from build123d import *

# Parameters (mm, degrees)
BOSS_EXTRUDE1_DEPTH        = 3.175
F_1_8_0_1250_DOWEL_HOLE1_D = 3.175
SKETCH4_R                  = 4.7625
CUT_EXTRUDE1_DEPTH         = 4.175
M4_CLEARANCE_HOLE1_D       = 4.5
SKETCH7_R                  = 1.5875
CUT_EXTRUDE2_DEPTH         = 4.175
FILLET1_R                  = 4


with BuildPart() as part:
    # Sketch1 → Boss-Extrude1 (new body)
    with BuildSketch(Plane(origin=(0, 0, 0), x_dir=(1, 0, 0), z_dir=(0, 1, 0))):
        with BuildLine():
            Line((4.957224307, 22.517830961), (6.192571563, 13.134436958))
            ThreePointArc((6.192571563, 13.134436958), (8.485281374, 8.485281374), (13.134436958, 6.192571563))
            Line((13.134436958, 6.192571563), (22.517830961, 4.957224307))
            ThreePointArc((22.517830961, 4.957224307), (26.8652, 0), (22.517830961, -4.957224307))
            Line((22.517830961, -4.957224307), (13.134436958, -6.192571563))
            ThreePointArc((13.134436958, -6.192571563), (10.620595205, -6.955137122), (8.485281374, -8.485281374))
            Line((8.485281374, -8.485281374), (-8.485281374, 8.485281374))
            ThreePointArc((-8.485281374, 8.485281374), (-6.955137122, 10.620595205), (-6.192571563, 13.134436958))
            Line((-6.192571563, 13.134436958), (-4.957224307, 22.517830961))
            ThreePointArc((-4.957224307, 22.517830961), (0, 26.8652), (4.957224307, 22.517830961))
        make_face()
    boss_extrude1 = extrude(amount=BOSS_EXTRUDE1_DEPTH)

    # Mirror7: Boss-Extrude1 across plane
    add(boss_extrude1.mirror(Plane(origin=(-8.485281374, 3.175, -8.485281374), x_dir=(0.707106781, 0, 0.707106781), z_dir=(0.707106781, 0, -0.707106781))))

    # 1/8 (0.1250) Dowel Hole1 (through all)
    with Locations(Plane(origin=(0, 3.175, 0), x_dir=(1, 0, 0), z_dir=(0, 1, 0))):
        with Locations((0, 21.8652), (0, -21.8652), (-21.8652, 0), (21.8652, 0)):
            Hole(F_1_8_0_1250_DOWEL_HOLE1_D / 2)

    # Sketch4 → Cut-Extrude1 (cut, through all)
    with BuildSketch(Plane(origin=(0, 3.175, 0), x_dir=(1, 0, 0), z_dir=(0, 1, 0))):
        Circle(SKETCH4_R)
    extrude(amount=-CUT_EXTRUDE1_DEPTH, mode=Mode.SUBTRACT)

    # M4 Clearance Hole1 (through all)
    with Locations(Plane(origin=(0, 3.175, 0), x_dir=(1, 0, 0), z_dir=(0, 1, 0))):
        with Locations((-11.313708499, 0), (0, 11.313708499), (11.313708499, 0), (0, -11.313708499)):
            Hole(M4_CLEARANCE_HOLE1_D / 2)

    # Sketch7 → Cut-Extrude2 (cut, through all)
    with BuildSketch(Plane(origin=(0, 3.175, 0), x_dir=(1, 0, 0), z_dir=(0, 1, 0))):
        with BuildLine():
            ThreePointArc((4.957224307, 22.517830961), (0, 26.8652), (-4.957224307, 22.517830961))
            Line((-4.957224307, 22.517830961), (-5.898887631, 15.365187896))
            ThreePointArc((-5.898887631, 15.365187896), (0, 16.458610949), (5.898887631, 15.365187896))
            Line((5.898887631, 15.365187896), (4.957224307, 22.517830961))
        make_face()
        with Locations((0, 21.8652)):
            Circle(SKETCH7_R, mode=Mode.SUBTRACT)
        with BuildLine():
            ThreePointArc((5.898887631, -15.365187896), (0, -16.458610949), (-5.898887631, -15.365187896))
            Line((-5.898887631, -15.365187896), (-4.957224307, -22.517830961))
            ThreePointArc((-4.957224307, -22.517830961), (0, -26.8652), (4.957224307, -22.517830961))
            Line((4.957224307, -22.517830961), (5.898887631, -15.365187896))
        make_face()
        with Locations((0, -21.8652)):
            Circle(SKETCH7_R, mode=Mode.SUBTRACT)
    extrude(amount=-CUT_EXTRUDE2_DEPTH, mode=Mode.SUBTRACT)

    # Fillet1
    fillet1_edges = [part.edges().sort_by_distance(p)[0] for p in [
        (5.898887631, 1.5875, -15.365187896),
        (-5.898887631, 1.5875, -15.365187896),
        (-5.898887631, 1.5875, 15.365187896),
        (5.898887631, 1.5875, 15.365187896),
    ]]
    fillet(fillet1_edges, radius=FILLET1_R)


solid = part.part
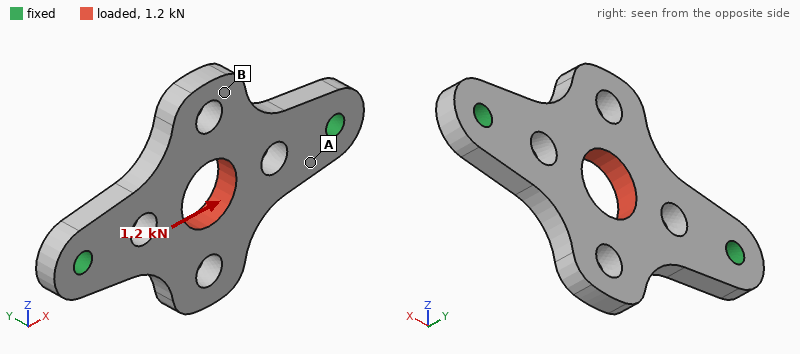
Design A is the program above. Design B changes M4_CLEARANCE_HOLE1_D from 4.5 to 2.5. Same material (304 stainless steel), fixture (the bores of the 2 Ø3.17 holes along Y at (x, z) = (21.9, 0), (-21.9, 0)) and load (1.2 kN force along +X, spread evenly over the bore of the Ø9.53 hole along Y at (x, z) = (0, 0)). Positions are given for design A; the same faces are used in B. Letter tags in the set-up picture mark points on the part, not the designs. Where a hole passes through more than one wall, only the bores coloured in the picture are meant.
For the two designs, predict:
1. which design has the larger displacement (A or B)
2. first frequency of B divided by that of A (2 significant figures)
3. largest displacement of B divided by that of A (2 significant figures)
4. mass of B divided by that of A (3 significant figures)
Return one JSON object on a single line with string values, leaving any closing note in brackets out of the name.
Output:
{"which design has the larger displacement": "A", "first frequency of B divided by that of A": "1.0", "largest displacement of B divided by that of A": "0.91", "mass of B divided by that of A": "1.06"}
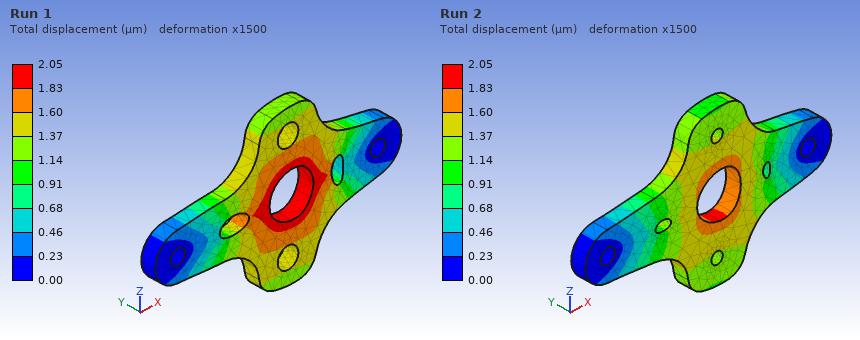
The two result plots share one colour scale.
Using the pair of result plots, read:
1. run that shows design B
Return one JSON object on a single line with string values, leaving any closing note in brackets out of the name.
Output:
{"run that shows design B": "Run 2"}
